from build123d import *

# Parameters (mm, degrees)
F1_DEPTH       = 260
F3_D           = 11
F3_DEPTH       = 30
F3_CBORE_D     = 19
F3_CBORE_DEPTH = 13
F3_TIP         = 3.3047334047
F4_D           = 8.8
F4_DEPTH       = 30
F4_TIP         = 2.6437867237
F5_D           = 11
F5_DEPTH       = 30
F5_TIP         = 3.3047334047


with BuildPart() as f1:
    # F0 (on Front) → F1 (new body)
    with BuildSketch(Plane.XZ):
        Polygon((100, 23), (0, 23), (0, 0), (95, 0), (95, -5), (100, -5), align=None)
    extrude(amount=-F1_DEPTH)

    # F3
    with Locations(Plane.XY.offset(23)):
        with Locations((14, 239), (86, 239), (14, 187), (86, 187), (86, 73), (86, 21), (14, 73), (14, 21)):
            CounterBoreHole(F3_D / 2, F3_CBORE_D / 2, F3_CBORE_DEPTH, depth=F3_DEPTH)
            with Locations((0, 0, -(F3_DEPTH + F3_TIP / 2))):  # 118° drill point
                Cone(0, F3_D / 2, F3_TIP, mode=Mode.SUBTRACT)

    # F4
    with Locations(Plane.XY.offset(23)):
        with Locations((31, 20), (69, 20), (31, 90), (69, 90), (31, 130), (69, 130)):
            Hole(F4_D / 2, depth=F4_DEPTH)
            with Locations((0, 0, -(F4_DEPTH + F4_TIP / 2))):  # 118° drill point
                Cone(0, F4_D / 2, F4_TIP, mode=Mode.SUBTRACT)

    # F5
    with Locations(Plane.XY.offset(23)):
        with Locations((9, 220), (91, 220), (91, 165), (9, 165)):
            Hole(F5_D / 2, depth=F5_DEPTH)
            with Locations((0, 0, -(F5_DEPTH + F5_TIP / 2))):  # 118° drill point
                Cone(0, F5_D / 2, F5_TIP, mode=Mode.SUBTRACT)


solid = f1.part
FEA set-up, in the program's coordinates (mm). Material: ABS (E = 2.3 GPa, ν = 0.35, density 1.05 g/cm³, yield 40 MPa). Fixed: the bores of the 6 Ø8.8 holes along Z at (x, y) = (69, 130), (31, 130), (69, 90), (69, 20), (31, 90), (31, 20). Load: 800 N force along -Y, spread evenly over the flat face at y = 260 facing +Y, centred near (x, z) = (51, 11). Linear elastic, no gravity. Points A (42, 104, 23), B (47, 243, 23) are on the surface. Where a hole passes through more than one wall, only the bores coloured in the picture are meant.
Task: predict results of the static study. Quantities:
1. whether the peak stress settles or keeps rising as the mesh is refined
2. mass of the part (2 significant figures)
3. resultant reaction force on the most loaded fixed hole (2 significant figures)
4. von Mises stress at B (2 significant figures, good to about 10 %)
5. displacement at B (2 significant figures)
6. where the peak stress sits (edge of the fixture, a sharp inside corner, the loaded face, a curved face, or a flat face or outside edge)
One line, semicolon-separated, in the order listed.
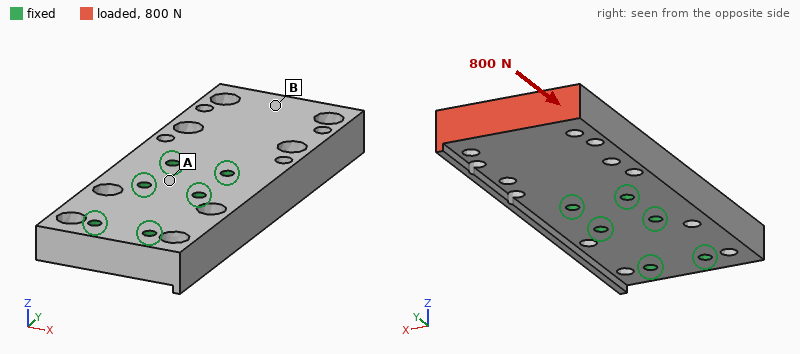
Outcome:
keeps rising; 580 g; 330 N; 0.34 MPa; 24 µm; a sharp inside corner
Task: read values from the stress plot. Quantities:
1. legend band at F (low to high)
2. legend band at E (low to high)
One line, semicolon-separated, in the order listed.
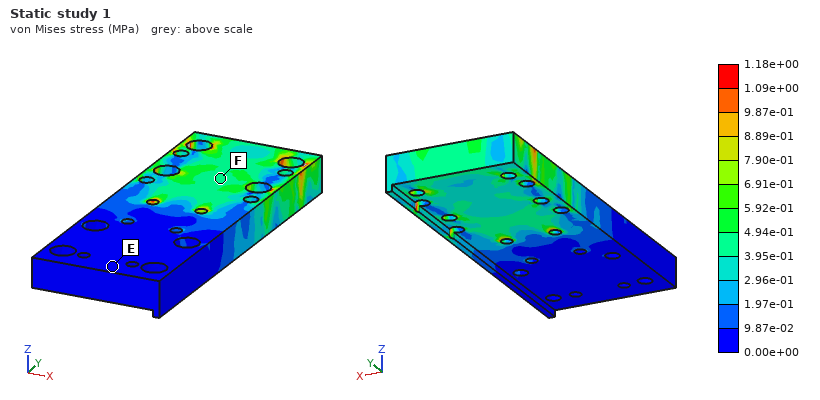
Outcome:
3.95e-01 to 4.94e-01 MPa; 0.00e+00 to 9.87e-02 MPa
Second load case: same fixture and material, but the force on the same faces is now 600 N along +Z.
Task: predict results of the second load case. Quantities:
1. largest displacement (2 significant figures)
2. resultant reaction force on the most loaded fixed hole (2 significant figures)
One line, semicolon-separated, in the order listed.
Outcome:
2.2 mm; 650 N
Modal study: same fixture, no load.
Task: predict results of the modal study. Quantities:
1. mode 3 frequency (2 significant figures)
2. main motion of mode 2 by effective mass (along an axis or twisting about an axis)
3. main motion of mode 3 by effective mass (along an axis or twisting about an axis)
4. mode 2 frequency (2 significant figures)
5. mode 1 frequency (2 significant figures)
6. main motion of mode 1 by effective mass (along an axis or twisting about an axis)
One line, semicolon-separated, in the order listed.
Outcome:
850 Hz; twisting about Y; along X; 800 Hz; 310 Hz; along Z
